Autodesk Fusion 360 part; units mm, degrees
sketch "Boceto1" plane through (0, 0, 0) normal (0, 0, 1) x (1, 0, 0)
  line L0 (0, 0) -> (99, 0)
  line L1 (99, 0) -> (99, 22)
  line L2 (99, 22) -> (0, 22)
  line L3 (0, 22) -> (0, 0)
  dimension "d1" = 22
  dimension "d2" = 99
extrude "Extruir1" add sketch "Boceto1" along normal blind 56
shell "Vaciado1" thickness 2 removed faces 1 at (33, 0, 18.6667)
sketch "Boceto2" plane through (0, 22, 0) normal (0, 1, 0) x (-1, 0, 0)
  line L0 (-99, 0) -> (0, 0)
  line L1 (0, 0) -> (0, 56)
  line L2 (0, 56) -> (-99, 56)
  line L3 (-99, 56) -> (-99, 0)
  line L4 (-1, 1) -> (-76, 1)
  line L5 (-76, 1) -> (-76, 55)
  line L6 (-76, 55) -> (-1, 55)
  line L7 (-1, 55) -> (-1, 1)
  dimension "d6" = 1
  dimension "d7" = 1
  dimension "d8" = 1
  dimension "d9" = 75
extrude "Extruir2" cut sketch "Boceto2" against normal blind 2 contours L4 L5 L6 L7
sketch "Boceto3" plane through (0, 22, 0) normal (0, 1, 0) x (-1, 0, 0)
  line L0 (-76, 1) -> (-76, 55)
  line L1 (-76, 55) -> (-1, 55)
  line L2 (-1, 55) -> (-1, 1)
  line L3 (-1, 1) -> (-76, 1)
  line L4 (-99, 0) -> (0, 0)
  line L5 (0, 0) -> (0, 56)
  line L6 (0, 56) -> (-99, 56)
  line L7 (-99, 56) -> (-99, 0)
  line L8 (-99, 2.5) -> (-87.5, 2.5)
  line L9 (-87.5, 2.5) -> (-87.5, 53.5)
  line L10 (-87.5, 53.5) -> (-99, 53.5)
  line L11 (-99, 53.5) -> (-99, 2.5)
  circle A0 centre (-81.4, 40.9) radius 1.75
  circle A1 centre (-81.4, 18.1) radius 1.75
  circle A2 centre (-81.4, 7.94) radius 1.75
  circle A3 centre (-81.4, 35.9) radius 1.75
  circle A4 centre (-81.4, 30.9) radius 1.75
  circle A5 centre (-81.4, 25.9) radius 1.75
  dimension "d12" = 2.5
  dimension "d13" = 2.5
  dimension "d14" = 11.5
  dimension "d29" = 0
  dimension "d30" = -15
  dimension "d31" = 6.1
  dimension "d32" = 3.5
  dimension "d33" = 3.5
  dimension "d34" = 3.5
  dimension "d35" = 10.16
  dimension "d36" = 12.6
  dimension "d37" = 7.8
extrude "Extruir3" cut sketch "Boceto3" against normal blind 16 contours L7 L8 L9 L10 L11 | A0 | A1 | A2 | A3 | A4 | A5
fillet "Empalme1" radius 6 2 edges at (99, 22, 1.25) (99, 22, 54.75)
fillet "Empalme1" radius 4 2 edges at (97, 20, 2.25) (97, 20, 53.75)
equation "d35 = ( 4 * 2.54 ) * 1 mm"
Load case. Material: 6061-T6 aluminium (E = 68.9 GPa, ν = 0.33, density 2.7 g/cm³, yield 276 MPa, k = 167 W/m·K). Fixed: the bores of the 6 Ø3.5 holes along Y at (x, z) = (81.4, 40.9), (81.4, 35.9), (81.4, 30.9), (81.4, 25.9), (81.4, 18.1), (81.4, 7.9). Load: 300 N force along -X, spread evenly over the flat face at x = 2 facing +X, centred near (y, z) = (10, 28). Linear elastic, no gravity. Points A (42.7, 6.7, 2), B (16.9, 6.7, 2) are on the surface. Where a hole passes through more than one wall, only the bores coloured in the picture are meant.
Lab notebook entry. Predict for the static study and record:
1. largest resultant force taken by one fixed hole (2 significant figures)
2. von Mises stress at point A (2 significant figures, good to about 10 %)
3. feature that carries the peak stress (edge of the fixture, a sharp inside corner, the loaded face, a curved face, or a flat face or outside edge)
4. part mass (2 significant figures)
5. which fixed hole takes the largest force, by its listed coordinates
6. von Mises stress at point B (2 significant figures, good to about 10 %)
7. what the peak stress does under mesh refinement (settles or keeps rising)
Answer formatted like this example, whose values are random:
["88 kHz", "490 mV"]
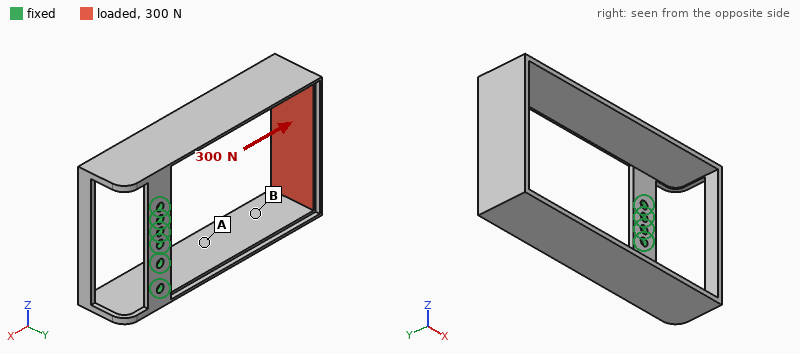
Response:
["310 N", "19 MPa", "edge of the fixture", "33 g", "(81.4, 40.9)", "45 MPa", "keeps rising"]
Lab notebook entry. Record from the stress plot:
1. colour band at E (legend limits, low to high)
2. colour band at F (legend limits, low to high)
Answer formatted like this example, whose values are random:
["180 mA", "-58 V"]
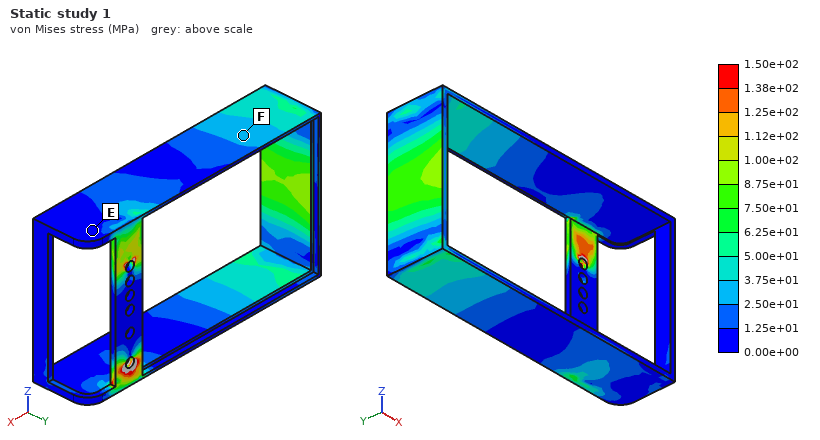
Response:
["0.00e+00 to 1.25e+01 MPa", "2.50e+01 to 3.75e+01 MPa"]
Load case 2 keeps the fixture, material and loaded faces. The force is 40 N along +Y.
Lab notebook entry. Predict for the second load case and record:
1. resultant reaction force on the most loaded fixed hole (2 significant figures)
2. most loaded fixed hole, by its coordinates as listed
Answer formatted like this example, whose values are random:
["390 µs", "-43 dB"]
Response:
["28 N", "(81.4, 40.9)"]
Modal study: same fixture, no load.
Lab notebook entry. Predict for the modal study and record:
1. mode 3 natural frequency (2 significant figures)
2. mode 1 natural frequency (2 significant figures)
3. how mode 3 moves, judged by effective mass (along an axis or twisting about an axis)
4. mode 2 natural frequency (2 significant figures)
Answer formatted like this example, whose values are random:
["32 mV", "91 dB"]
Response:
["560 Hz", "250 Hz", "twisting about X", "260 Hz"]
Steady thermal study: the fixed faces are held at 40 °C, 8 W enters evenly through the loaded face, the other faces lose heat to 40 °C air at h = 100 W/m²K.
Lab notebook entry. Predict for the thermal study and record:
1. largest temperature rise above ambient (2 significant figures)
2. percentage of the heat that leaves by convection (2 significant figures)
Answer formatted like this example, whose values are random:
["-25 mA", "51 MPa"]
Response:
["19 K", "92 %"]
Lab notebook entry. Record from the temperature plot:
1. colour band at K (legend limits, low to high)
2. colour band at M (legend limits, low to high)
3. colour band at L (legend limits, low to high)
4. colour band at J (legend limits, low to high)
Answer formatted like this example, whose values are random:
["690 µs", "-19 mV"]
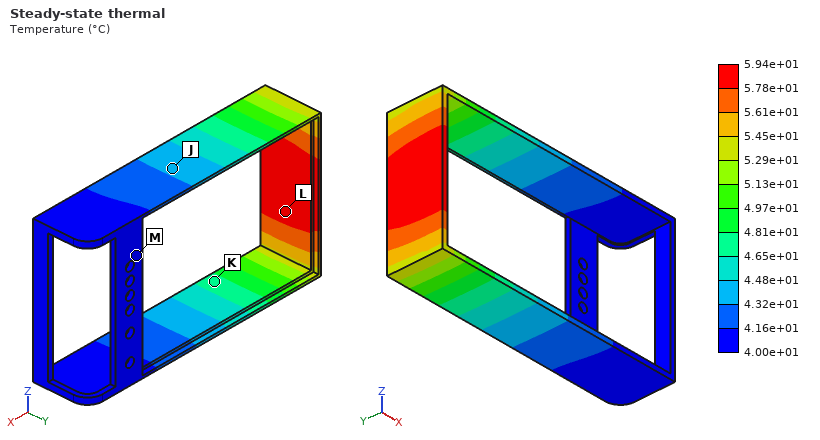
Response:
["4.65e+01 to 4.81e+01 °C", "4.00e+01 to 4.16e+01 °C", "5.78e+01 to 5.94e+01 °C", "4.32e+01 to 4.48e+01 °C"]
